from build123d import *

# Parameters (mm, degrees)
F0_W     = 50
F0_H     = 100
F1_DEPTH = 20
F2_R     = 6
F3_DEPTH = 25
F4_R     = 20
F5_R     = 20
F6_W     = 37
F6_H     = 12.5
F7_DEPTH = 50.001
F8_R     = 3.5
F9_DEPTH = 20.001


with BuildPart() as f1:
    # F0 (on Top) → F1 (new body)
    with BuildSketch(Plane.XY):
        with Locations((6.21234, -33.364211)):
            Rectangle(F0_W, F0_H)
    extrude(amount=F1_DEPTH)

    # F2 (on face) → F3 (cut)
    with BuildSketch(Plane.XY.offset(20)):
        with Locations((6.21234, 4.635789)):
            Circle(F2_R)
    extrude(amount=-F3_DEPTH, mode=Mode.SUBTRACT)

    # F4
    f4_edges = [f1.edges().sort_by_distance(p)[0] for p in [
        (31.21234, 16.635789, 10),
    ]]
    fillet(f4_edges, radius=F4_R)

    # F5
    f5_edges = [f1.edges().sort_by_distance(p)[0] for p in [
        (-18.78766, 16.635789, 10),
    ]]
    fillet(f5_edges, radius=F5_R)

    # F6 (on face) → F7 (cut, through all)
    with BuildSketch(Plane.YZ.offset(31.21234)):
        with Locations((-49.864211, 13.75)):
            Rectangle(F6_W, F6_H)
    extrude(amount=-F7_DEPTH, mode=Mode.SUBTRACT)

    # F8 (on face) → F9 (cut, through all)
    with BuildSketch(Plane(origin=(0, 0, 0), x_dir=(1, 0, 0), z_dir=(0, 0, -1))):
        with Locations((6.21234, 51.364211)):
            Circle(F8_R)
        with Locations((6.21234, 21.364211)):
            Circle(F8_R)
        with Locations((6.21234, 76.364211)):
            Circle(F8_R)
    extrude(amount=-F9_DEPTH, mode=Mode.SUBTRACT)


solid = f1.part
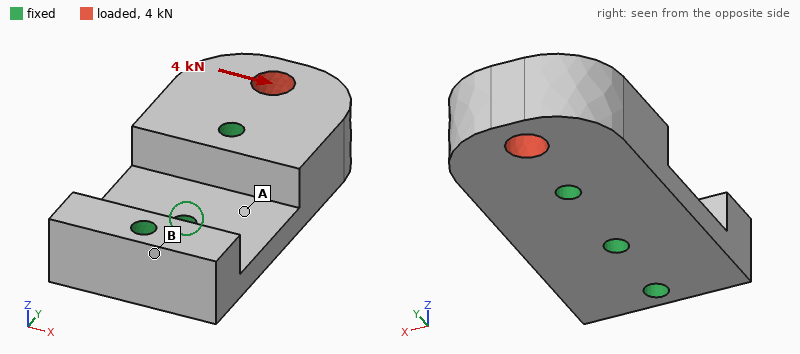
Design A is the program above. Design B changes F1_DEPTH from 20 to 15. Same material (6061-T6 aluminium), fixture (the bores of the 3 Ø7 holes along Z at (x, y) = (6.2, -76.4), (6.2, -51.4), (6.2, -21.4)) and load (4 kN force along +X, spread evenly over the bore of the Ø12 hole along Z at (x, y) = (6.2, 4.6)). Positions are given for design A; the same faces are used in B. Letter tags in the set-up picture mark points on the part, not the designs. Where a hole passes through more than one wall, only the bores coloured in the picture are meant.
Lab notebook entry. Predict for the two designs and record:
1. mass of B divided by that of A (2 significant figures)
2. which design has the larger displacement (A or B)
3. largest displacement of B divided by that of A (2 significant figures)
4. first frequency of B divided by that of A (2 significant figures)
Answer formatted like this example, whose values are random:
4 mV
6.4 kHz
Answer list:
0.80
B
1.2
0.85
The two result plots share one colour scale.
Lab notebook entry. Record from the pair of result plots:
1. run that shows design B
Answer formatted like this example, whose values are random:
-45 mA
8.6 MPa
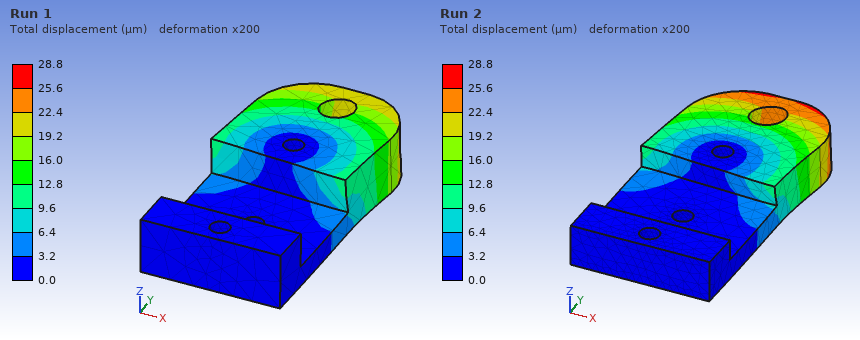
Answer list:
Run 2
